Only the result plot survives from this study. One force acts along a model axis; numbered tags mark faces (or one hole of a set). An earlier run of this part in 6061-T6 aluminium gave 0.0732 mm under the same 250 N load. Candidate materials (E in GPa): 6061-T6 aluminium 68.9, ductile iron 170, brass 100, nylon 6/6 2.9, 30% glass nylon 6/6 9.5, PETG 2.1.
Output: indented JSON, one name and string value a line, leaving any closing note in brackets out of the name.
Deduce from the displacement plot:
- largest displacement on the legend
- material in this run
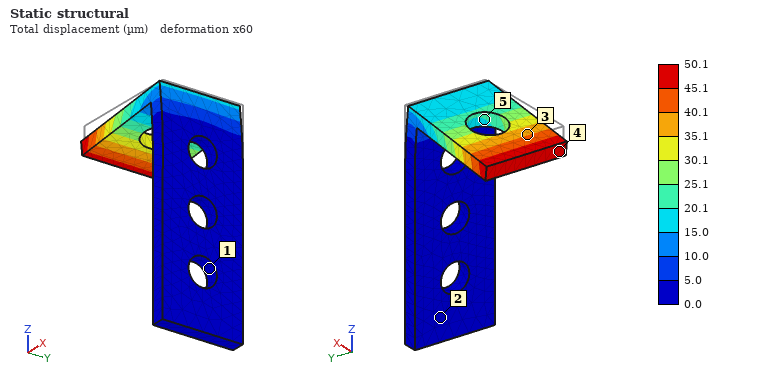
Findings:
{
  "largest displacement on the legend": "50.1 µm",
  "material in this run": "brass"
}
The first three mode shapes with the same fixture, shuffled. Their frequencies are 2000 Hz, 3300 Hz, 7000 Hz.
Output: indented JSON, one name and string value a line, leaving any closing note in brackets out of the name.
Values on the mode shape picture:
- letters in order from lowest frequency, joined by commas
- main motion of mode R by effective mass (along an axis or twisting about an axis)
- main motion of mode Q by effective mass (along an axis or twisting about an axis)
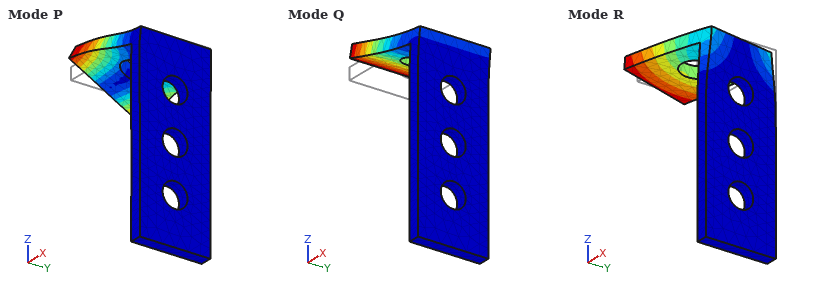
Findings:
{
  "letters in order from lowest frequency, joined by commas": "Q, R, P",
  "main motion of mode R by effective mass": "along Y",
  "main motion of mode Q by effective mass": "along Z"
}
